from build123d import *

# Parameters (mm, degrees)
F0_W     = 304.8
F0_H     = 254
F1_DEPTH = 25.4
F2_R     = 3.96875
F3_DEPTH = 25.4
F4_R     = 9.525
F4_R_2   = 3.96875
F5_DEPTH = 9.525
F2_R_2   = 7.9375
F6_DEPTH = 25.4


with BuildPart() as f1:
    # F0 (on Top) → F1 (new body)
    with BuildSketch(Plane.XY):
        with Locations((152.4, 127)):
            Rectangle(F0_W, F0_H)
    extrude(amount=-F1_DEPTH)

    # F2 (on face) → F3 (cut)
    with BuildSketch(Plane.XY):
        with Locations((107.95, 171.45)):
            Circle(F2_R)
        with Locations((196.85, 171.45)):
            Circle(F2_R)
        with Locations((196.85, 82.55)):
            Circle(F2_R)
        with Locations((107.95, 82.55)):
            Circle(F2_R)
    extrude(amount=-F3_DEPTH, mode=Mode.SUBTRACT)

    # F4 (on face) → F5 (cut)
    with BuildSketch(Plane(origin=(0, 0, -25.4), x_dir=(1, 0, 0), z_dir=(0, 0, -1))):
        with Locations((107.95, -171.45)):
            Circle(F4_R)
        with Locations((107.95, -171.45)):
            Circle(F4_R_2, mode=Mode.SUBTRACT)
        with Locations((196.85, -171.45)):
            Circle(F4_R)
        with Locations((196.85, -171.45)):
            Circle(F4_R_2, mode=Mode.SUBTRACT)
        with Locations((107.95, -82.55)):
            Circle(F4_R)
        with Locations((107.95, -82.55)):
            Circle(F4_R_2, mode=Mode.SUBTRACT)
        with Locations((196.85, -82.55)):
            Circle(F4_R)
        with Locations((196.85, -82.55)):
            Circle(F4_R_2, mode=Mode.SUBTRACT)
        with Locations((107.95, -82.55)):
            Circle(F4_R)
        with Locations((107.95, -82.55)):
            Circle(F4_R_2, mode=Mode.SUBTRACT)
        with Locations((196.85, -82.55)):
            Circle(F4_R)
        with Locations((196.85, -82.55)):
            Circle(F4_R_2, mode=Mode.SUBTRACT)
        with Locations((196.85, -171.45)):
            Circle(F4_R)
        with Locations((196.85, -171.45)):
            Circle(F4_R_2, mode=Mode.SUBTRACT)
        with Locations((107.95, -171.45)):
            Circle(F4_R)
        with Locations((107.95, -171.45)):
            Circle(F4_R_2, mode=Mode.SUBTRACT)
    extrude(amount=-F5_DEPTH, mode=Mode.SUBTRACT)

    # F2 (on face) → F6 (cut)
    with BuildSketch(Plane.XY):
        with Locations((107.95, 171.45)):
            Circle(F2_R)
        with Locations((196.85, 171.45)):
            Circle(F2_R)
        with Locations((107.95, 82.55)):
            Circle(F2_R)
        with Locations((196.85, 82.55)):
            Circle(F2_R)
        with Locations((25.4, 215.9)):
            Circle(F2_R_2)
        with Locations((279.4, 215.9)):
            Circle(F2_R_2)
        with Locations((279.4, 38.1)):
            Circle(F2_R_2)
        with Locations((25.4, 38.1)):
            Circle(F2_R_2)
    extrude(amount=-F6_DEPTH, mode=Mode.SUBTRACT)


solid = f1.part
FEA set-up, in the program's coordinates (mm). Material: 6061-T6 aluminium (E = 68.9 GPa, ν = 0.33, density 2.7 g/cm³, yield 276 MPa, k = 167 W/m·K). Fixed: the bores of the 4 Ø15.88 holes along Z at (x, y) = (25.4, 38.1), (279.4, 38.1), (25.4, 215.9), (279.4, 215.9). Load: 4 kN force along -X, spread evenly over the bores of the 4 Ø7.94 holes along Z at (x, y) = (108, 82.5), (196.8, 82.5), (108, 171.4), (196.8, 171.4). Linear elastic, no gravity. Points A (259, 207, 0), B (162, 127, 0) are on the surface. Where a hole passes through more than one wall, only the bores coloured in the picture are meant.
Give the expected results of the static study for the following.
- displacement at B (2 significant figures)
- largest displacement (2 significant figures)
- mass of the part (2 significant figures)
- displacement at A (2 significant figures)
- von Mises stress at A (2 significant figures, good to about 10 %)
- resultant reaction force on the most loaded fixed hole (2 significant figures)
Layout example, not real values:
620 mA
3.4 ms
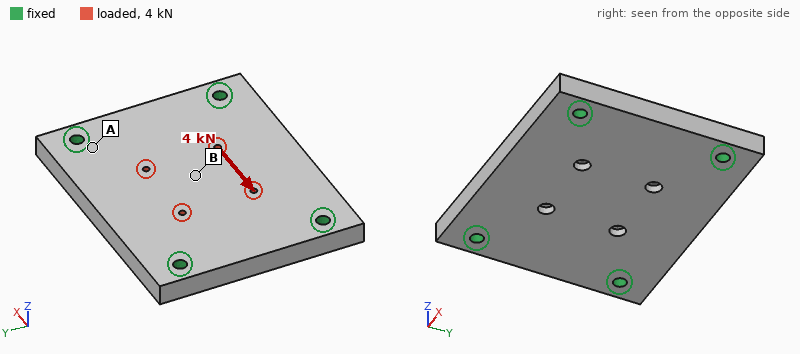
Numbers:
0.96 µm
1.4 µm
5.2 kg
0.22 µm
0.90 MPa
1.0 kN
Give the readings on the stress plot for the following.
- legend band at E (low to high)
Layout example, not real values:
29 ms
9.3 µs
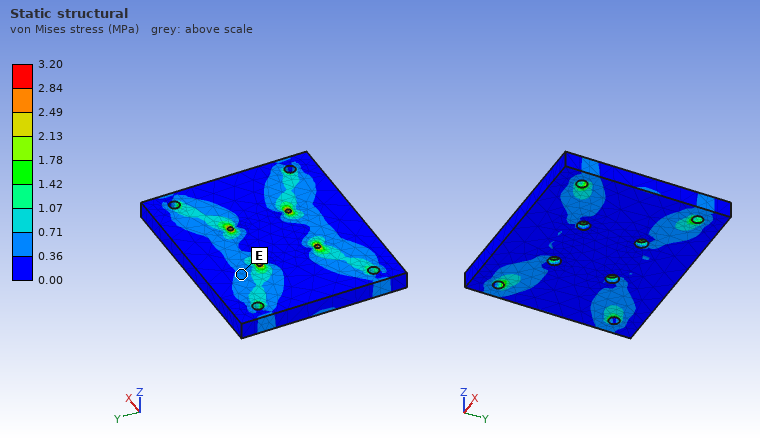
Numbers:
0.36 to 0.71 MPa
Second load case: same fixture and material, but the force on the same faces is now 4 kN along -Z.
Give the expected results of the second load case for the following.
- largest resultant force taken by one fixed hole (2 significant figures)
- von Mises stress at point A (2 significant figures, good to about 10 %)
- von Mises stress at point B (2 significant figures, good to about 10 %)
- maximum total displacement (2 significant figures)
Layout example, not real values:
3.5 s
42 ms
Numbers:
1.0 kN
3.9 MPa
2.7 MPa
20 µm
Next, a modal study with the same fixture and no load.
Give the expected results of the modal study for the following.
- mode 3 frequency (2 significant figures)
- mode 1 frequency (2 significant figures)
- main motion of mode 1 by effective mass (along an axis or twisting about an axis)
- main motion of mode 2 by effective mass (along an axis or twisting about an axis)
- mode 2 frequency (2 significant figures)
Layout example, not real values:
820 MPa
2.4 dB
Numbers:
3000 Hz
1600 Hz
along Z
twisting about X
2200 Hz
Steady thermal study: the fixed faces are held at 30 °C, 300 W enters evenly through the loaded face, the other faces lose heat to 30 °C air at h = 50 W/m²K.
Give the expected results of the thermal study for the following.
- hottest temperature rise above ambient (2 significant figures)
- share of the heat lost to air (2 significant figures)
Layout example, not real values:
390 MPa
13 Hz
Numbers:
21 K
24 %
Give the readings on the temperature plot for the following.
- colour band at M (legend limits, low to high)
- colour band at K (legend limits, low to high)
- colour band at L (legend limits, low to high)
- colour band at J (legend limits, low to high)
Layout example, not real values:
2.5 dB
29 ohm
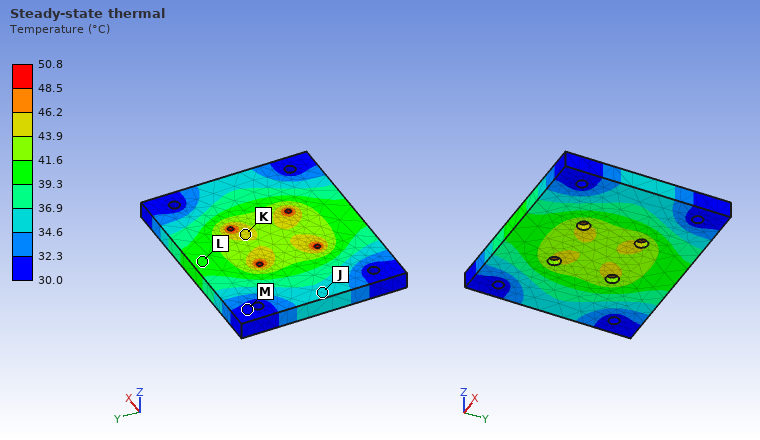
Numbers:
30.0 to 32.3 °C
43.9 to 46.2 °C
39.3 to 41.6 °C
34.6 to 36.9 °C
